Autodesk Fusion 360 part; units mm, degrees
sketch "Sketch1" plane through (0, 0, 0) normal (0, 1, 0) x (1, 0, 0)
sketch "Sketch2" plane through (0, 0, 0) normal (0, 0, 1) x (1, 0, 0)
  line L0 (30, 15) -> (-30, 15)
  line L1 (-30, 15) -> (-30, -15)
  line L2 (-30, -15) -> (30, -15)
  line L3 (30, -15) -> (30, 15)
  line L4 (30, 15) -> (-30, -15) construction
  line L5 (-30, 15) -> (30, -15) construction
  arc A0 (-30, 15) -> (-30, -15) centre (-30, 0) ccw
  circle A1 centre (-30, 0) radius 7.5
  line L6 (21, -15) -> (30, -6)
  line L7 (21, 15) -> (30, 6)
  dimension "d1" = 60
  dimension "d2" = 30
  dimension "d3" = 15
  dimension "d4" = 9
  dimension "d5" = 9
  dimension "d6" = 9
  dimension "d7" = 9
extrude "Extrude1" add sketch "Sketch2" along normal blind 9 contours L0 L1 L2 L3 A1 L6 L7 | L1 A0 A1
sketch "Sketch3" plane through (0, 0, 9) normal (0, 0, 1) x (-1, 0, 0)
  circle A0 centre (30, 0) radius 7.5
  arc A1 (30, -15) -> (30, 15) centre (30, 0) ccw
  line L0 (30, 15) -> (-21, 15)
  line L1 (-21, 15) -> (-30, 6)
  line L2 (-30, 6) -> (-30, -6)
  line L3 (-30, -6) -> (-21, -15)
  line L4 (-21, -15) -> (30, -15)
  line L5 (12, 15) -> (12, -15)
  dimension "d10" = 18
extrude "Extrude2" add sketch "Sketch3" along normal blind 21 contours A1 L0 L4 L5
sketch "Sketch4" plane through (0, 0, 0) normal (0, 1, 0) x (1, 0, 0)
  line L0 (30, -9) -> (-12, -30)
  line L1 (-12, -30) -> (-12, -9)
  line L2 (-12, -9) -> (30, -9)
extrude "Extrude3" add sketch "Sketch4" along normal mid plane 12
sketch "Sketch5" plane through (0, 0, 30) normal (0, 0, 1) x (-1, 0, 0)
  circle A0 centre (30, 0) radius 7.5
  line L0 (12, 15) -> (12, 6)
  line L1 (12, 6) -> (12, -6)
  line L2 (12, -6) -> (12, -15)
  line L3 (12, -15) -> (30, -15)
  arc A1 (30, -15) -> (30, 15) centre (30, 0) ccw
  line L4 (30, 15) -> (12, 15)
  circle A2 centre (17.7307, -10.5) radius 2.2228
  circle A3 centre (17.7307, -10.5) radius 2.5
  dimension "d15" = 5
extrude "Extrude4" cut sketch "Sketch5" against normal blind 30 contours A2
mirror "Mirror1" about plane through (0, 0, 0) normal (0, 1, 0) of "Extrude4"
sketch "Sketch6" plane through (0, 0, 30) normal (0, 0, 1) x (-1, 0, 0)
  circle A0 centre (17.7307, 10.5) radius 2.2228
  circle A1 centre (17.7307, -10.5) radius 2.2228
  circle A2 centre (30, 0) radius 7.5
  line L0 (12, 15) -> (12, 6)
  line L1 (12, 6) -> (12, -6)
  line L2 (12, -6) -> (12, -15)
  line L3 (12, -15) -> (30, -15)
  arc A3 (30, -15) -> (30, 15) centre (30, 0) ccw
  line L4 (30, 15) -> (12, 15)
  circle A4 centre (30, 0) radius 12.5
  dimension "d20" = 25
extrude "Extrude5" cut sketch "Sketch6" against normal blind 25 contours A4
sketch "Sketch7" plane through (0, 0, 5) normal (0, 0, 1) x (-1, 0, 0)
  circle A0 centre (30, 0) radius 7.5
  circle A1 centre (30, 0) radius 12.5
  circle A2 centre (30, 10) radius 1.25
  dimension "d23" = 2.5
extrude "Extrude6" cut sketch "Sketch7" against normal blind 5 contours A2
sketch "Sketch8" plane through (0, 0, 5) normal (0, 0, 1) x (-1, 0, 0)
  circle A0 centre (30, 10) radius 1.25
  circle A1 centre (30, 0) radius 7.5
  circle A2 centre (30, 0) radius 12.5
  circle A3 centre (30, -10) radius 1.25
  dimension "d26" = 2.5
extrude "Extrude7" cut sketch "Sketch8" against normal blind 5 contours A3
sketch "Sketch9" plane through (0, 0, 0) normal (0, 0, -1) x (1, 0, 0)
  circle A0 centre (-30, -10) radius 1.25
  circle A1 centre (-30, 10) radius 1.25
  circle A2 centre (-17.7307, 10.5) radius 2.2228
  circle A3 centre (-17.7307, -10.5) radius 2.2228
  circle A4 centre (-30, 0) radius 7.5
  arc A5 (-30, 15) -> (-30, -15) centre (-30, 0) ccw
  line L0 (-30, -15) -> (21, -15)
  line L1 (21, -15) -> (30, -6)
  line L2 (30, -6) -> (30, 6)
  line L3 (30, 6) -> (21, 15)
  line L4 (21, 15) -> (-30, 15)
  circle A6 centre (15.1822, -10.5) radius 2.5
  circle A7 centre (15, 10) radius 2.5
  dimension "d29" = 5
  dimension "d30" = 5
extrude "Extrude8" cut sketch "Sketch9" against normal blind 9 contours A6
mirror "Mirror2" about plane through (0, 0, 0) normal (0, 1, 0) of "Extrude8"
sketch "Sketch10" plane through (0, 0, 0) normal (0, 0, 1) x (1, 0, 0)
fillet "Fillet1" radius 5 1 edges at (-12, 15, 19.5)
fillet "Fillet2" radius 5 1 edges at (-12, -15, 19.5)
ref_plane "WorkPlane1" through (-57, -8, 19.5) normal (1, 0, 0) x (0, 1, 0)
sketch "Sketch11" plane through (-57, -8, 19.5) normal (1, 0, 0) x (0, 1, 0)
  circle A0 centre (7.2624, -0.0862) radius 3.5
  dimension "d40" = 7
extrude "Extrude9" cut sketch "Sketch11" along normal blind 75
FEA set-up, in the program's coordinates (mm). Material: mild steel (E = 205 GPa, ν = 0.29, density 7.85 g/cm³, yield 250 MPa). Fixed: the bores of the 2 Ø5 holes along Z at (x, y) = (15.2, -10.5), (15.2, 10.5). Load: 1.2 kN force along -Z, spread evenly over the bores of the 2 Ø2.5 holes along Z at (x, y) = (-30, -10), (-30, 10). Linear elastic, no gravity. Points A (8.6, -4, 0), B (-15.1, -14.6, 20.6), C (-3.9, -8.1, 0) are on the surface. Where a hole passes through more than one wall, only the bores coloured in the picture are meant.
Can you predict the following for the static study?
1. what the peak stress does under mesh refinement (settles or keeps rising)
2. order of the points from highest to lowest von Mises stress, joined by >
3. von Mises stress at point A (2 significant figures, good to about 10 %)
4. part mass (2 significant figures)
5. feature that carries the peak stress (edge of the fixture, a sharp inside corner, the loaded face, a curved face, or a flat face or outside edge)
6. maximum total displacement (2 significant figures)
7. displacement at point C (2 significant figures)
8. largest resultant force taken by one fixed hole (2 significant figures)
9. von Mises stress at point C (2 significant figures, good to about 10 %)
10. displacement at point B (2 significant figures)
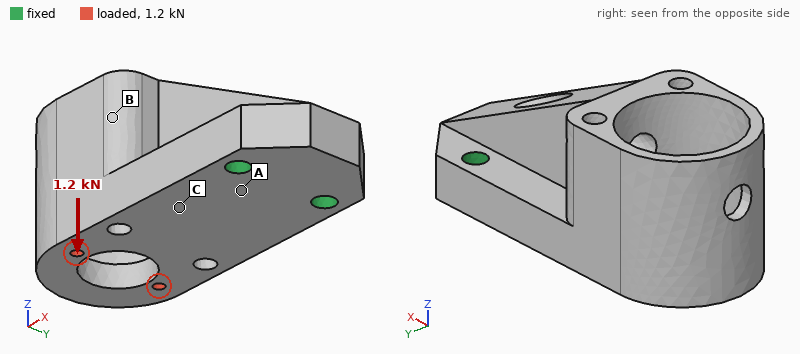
keeps rising
A > C > B
46 MPa
210 g
edge of the fixture
65 µm
15 µm
700 N
23 MPa
30 µm
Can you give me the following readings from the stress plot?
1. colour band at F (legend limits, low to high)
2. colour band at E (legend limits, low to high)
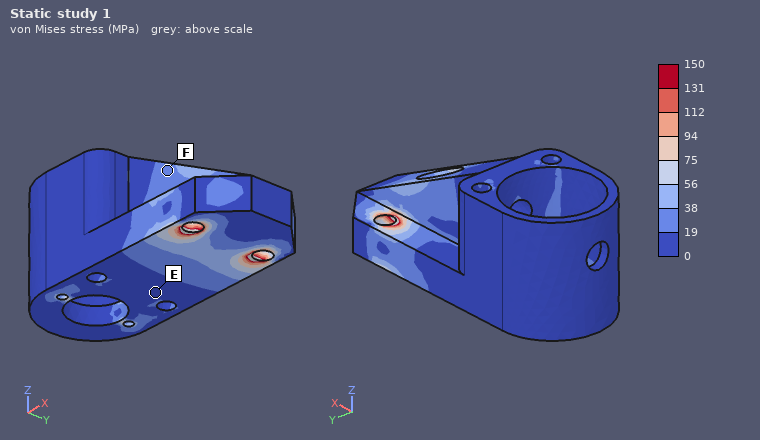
19 to 38 MPa
0 to 19 MPa
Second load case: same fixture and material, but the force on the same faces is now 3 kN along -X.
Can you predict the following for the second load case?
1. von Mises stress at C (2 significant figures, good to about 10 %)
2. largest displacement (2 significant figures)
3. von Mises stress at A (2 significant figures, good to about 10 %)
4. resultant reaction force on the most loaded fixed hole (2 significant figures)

16 MPa
15 µm
15 MPa
1.5 kN
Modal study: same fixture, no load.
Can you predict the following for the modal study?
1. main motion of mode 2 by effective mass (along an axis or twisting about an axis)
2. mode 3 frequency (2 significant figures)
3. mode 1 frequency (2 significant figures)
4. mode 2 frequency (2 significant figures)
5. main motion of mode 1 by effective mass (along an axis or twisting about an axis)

along Y
7300 Hz
2700 Hz
4900 Hz
along Z
